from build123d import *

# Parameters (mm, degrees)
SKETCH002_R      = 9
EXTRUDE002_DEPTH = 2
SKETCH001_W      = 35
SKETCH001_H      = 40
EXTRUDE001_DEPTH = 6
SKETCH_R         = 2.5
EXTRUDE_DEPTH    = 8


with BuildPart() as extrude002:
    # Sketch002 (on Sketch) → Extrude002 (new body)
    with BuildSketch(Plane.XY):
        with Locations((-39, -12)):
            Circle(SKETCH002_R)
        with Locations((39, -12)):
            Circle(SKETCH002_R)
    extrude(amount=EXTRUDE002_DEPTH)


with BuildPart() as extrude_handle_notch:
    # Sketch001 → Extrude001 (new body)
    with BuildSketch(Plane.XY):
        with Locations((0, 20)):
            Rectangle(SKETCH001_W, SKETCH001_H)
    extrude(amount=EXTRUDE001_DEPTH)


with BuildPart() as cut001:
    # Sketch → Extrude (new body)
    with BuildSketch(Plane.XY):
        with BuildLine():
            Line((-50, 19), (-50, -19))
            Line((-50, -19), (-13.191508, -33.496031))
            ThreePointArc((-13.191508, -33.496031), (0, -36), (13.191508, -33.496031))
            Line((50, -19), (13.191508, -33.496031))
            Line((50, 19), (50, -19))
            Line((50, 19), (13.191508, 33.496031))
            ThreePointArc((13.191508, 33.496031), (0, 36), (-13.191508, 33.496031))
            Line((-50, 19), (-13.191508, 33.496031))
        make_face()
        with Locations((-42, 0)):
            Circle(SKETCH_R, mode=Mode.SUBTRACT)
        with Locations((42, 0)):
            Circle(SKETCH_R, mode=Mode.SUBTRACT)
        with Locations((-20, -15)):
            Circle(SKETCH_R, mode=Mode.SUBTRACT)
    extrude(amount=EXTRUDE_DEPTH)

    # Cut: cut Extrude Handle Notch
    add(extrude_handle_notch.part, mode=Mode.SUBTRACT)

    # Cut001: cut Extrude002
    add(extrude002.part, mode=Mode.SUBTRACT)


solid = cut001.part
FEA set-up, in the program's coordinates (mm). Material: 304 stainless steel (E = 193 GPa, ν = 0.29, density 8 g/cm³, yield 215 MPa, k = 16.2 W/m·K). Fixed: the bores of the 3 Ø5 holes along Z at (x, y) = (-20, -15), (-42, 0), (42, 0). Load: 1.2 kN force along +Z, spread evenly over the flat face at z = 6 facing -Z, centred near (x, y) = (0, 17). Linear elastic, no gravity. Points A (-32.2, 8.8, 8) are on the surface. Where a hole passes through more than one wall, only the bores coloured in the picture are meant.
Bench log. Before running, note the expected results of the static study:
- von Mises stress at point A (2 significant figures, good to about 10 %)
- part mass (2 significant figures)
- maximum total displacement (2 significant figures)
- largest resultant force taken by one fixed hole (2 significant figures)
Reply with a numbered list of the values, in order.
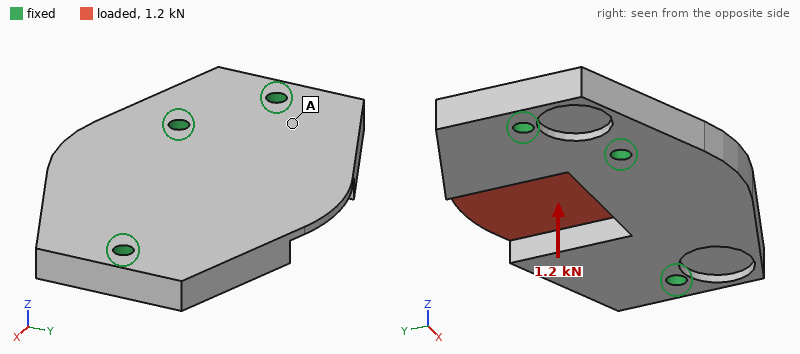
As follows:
1. 21 MPa
2. 300 g
3. 95 µm
4. 800 N
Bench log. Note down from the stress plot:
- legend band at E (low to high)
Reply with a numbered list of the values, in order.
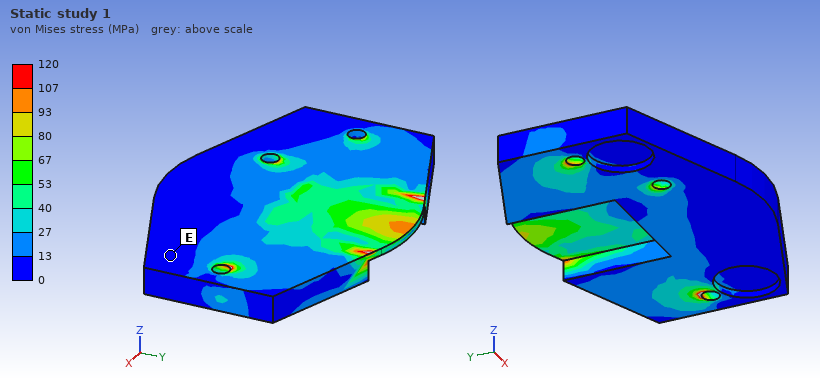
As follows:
1. 0 to 13 MPa
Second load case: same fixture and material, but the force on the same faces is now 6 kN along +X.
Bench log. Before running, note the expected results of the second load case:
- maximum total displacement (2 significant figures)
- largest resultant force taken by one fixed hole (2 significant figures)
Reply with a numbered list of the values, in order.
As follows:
1. 22 µm
2. 2.8 kN
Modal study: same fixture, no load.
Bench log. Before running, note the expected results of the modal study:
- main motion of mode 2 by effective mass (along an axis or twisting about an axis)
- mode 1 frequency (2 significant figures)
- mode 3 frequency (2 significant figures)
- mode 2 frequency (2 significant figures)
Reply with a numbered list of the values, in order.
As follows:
1. along Z
2. 4500 Hz
3. 6300 Hz
4. 5900 Hz
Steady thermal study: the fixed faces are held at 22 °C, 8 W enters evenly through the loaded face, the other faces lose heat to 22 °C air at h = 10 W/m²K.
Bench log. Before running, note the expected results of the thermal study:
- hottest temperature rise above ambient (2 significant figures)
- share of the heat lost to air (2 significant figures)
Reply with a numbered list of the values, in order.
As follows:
1. 55 K
2. 17 %
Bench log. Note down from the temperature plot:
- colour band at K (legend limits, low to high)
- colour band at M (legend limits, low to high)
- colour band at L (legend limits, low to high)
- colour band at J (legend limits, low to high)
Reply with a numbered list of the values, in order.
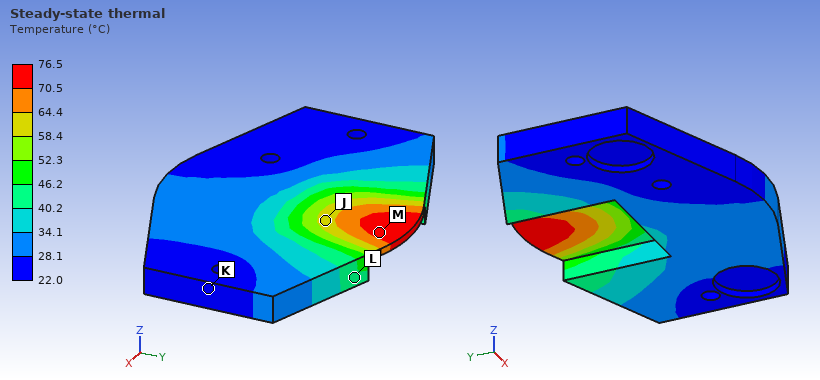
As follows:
1. 22.0 to 28.1 °C
2. 70.5 to 76.5 °C
3. 40.2 to 46.2 °C
4. 58.4 to 64.4 °C
